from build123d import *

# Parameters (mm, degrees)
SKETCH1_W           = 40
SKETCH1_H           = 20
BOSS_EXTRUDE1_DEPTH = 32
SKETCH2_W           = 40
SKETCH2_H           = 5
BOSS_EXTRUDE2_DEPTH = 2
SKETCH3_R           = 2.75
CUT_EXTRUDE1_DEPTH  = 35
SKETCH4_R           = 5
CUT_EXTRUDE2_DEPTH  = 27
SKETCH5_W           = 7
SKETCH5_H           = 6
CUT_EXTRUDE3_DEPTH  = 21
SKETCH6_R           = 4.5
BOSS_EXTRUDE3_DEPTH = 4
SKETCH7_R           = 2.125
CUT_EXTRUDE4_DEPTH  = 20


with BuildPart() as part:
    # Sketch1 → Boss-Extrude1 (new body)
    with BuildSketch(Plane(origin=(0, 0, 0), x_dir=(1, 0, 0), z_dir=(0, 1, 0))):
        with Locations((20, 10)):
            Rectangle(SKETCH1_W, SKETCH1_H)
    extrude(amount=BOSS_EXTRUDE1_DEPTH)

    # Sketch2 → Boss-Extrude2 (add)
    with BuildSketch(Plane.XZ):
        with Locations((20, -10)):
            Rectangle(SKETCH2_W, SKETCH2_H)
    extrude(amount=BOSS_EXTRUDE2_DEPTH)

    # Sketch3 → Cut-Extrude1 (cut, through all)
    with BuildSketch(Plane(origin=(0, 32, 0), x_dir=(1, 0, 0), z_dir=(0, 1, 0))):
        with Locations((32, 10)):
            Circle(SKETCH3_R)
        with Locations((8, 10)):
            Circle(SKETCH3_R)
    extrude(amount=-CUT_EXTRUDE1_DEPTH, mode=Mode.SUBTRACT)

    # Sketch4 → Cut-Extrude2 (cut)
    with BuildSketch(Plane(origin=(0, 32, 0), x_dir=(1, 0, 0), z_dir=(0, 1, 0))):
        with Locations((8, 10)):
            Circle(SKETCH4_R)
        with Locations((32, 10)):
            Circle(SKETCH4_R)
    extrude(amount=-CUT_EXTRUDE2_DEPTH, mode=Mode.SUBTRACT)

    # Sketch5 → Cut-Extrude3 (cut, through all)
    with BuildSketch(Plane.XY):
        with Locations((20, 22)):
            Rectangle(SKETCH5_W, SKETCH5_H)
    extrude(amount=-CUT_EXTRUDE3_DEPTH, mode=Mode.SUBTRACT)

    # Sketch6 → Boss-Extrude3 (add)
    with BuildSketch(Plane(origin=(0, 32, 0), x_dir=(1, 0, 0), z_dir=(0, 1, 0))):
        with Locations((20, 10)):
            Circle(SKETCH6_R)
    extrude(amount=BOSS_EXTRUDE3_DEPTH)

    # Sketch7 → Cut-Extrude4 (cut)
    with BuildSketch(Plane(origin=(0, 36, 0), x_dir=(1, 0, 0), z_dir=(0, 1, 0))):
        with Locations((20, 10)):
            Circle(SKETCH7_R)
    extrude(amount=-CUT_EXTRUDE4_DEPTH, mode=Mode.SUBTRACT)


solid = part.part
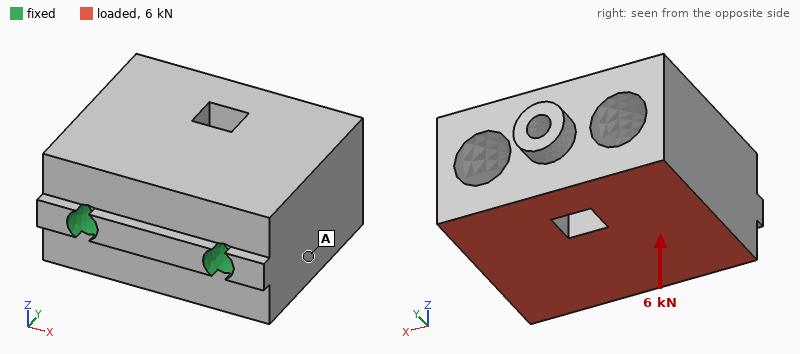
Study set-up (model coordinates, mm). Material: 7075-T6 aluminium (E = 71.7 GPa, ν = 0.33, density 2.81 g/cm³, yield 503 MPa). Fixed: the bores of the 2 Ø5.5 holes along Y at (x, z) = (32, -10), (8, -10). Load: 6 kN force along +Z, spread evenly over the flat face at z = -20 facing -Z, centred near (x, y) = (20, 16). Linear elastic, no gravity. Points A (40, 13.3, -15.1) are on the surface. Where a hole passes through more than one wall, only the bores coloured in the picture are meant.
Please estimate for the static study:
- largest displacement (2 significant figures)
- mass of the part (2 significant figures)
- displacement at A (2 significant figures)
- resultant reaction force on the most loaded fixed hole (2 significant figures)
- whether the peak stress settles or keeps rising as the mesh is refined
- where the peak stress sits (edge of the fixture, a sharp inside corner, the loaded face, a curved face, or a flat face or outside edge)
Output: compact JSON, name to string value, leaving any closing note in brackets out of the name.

{"largest displacement": "0.14 mm", "mass of the part": "58 g", "displacement at A": "0.049 mm", "resultant reaction force on the most loaded fixed hole": "3.0 kN", "whether the peak stress settles or keeps rising as the mesh is refined": "keeps rising", "where the peak stress sits": "edge of the fixture"}
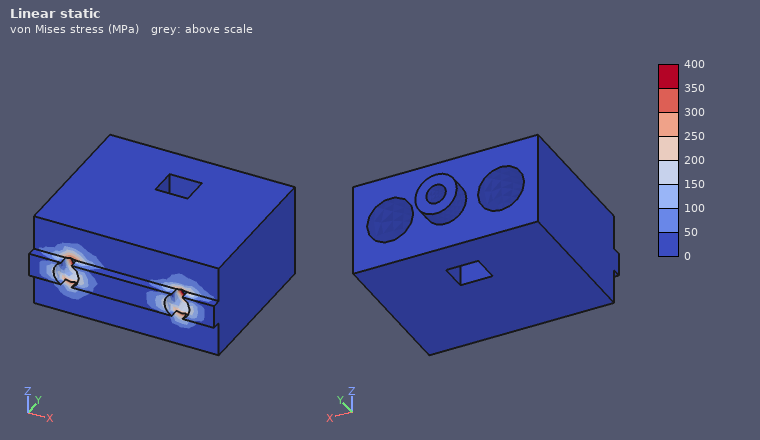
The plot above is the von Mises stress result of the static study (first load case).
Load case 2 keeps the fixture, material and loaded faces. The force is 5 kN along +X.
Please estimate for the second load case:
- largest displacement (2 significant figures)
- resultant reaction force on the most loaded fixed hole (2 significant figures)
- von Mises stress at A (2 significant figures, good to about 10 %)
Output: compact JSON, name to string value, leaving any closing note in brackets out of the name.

{"largest displacement": "29 µm", "resultant reaction force on the most loaded fixed hole": "3.9 kN", "von Mises stress at A": "15 MPa"}
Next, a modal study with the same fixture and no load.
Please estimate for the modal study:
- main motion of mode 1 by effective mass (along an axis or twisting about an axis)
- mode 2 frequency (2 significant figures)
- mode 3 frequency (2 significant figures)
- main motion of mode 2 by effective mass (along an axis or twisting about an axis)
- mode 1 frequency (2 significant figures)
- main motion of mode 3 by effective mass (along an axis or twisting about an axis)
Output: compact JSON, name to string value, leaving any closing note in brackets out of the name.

{"main motion of mode 1 by effective mass": "along Z", "mode 2 frequency": "12 kHz", "mode 3 frequency": "16 kHz", "main motion of mode 2 by effective mass": "along X", "mode 1 frequency": "5400 Hz", "main motion of mode 3 by effective mass": "twisting about Y"}
